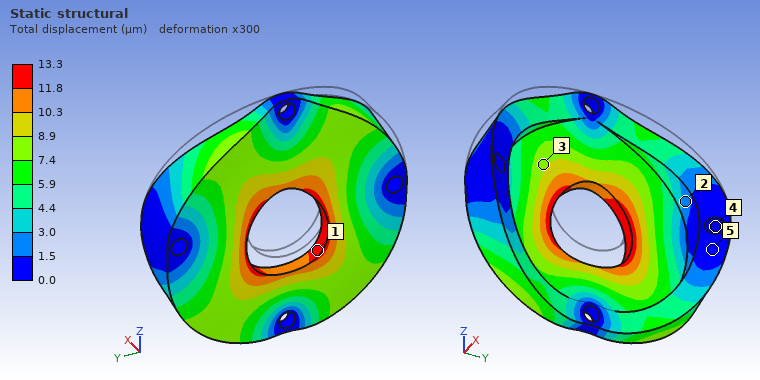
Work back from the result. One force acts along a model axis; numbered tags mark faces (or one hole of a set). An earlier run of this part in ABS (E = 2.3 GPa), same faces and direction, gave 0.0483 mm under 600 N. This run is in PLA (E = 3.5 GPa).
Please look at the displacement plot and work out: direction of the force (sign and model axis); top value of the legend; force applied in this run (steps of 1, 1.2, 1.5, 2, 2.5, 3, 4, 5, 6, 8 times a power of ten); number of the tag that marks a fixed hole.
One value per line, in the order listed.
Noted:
-Z
13.3 µm
250 N
4
